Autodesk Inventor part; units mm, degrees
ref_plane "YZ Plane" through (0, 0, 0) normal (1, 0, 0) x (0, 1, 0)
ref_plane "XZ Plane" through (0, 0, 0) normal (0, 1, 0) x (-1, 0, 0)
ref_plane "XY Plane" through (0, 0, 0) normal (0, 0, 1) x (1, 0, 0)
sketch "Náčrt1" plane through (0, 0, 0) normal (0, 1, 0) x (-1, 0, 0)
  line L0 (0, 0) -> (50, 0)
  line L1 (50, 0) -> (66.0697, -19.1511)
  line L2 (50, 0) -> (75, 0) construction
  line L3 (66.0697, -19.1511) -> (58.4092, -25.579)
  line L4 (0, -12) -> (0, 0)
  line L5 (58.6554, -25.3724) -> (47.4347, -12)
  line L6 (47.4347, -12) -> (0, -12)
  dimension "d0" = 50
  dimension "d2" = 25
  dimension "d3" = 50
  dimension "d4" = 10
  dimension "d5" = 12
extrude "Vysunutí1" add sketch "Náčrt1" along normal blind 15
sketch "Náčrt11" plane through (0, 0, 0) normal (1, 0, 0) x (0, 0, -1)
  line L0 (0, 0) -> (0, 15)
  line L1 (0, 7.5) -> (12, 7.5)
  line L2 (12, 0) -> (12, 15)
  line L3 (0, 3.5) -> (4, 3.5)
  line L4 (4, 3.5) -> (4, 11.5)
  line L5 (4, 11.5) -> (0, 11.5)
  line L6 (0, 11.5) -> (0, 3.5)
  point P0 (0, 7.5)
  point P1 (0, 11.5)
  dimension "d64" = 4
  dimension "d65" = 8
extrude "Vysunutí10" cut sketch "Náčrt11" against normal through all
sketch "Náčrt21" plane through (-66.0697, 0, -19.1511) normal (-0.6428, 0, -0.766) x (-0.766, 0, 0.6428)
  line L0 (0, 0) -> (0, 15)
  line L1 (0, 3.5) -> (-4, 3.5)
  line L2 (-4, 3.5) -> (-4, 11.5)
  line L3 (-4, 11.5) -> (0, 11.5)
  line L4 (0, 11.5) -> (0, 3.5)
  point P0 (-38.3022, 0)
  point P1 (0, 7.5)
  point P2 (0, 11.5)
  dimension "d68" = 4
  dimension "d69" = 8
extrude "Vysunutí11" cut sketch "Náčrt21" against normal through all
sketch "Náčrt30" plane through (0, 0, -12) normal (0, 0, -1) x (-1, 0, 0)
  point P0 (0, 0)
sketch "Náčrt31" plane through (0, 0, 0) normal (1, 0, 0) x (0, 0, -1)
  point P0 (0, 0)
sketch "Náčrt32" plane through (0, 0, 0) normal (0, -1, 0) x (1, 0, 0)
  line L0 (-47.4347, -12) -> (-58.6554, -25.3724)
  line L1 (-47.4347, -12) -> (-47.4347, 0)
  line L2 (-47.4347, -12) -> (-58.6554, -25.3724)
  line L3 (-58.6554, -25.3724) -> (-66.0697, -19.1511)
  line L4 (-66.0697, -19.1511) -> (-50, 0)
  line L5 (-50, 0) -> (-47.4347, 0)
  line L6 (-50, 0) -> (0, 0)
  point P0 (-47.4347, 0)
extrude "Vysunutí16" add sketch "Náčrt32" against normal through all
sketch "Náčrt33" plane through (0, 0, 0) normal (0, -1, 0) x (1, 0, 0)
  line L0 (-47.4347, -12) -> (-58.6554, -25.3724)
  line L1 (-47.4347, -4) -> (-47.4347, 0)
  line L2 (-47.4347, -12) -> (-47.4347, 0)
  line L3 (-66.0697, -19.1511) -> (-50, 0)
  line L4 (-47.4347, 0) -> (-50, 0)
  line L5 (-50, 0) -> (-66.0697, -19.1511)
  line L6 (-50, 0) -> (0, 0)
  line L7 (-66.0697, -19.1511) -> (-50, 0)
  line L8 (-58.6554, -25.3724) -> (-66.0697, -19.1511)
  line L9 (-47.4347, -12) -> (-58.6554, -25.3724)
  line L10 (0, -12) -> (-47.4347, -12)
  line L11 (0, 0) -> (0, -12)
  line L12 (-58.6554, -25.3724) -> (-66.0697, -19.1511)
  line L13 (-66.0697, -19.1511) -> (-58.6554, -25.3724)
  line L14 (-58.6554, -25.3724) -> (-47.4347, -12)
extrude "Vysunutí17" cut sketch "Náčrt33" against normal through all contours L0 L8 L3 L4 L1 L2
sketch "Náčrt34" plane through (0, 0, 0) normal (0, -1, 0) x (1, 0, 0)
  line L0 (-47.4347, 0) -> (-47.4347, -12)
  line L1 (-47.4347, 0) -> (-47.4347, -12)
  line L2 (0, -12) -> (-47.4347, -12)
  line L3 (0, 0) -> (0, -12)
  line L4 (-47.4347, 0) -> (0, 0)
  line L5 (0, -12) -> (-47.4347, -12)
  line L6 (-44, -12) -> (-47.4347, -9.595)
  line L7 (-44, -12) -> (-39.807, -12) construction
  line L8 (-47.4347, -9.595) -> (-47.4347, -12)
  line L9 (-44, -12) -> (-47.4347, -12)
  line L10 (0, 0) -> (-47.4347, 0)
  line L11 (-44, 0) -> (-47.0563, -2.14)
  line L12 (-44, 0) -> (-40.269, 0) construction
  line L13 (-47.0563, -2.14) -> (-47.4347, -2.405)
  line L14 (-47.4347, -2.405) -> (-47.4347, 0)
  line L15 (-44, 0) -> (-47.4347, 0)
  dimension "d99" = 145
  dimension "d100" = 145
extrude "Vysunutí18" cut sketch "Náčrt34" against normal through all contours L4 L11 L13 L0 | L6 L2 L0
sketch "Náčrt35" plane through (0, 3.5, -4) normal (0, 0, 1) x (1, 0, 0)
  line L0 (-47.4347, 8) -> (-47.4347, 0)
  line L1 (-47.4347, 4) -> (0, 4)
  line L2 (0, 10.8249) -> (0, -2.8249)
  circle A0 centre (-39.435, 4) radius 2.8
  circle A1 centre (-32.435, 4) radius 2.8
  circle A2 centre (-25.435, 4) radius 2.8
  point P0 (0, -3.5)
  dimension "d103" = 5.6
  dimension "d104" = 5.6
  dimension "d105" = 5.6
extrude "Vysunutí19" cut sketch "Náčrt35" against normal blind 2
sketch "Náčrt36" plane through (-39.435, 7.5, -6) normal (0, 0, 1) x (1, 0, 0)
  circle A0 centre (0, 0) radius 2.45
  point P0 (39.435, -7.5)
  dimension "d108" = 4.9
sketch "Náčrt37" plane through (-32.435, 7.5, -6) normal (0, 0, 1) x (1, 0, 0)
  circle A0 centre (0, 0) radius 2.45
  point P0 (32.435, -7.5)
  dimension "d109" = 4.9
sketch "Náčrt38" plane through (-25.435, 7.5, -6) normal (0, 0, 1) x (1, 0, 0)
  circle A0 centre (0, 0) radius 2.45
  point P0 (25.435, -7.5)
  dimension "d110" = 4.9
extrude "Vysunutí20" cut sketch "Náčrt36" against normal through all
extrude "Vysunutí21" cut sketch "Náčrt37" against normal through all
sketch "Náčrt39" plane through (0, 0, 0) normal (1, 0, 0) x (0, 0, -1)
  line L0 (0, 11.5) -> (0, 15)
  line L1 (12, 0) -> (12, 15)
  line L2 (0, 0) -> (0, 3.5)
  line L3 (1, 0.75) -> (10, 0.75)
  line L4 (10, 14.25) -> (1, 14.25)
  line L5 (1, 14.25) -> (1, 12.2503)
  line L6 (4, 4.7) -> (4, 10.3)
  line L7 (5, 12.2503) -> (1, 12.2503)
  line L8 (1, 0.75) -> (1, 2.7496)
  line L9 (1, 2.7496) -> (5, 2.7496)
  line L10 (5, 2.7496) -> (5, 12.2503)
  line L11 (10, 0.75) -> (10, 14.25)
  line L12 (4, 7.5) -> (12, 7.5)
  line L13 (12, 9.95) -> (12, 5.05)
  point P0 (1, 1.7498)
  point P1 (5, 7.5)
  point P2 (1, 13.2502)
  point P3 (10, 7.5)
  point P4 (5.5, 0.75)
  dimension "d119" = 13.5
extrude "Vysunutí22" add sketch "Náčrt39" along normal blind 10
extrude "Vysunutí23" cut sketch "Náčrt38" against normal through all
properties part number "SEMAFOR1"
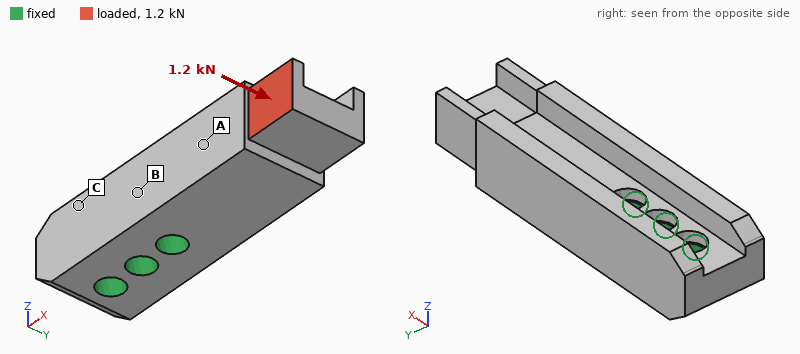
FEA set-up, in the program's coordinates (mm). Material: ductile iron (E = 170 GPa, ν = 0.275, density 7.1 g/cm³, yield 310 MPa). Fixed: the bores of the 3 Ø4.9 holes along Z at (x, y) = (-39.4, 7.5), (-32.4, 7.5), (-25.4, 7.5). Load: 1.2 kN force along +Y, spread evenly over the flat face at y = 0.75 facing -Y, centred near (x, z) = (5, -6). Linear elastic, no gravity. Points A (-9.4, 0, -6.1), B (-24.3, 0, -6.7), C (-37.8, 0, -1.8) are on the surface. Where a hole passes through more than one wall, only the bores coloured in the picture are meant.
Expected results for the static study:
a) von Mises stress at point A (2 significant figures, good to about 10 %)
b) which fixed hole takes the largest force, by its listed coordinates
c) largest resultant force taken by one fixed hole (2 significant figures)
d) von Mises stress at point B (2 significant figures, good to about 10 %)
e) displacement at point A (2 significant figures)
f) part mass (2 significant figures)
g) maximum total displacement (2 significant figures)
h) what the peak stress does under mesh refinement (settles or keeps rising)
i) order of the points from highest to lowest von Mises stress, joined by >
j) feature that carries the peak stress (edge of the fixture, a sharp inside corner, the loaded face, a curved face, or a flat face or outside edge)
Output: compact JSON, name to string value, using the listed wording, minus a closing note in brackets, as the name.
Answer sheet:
{"von Mises stress at point A": "48 MPa", "which fixed hole takes the largest force, by its listed coordinates": "(-25.4, 7.5)", "largest resultant force taken by one fixed hole": "2.8 kN", "von Mises stress at point B": "80 MPa", "displacement at point A": "20 µm", "part mass": "52 g", "maximum total displacement": "66 µm", "what the peak stress does under mesh refinement": "keeps rising", "order of the points from highest to lowest von Mises stress, joined by >": "B > A > C", "feature that carries the peak stress": "edge of the fixture"}
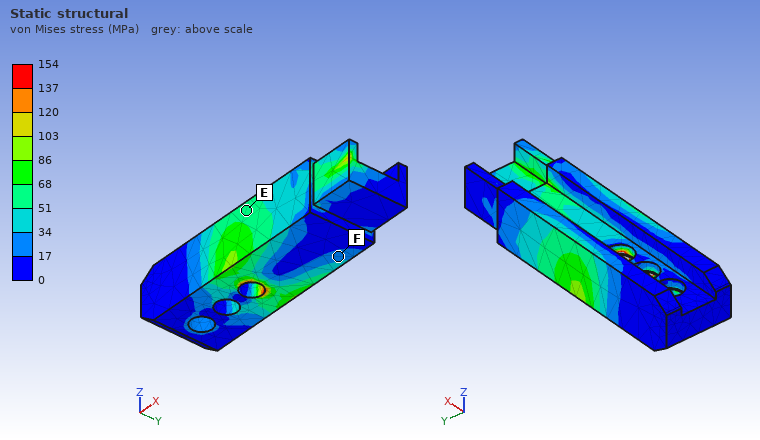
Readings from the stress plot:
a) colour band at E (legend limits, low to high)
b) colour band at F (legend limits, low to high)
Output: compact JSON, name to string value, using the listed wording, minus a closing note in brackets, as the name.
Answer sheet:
{"colour band at E": "51 to 68 MPa", "colour band at F": "17 to 34 MPa"}
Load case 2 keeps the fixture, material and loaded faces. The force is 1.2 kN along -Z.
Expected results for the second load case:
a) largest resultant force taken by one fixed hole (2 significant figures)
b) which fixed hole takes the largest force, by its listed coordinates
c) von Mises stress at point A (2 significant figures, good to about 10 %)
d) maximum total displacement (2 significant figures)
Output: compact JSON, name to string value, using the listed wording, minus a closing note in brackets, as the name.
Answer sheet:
{"largest resultant force taken by one fixed hole": "3.1 kN", "which fixed hole takes the largest force, by its listed coordinates": "(-25.4, 7.5)", "von Mises stress at point A": "67 MPa", "maximum total displacement": "0.10 mm"}
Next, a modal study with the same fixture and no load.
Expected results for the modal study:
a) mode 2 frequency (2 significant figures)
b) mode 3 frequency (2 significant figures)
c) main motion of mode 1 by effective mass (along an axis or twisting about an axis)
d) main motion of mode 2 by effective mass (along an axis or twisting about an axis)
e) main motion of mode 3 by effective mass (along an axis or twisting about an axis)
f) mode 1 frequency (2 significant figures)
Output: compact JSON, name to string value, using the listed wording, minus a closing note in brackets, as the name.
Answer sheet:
{"mode 2 frequency": "8300 Hz", "mode 3 frequency": "16 kHz", "main motion of mode 1 by effective mass": "along Z", "main motion of mode 2 by effective mass": "along Y", "main motion of mode 3 by effective mass": "twisting about X", "mode 1 frequency": "6800 Hz"}
